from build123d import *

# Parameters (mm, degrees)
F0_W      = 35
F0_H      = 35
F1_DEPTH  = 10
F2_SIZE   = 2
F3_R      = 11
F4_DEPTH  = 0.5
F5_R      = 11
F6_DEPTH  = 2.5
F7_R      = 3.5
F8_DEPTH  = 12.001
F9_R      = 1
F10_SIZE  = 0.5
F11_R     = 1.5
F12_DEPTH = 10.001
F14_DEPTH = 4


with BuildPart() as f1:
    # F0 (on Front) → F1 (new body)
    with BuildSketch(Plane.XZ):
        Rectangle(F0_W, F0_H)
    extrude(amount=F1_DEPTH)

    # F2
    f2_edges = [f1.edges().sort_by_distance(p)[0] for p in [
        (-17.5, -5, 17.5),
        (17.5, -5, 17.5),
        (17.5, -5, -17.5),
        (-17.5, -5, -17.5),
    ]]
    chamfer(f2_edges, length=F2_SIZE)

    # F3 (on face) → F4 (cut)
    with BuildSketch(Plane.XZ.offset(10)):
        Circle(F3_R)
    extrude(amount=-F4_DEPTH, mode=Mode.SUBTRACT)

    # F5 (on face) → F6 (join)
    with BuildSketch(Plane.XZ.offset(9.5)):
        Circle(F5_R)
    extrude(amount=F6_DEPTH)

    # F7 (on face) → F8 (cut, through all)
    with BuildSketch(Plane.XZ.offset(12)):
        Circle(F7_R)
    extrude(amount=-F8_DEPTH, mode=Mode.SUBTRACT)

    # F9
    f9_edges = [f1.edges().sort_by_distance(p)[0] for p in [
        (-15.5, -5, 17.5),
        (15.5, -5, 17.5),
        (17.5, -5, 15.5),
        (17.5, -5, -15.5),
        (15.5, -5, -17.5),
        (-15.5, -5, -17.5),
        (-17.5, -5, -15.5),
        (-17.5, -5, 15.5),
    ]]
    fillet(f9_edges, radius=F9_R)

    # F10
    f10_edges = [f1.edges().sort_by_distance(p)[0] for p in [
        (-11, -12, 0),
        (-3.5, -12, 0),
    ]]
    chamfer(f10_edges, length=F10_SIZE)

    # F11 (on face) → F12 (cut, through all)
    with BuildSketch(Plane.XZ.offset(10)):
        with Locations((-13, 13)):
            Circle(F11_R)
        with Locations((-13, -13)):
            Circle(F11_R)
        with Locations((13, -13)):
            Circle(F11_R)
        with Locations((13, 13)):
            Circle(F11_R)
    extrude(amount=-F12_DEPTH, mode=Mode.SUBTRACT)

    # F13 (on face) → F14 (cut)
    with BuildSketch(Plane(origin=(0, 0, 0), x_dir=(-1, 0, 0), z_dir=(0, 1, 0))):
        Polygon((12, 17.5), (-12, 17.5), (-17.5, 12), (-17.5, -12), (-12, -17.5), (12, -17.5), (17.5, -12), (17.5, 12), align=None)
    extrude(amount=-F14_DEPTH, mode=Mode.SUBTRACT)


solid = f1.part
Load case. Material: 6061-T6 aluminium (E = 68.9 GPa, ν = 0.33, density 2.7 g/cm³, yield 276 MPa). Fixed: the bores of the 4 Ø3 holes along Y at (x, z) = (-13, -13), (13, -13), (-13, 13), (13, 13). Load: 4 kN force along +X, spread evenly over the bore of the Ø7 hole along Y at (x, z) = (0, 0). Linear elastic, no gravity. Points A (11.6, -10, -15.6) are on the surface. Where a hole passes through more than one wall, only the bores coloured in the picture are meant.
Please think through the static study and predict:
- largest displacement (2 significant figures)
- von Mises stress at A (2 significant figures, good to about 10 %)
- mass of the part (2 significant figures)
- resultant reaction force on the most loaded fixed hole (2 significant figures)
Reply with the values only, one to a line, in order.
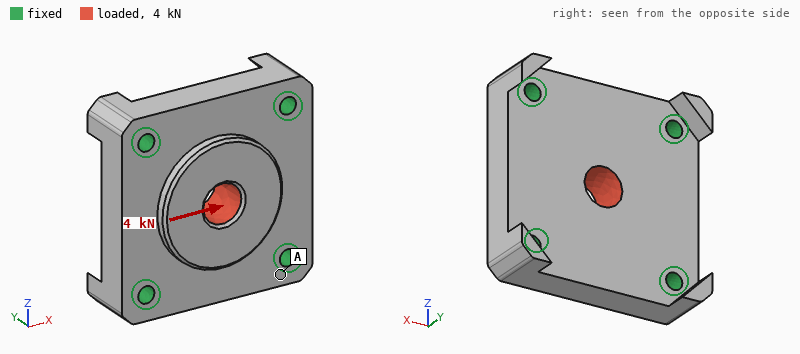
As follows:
5.9 µm
7.6 MPa
21 g
1.1 kN
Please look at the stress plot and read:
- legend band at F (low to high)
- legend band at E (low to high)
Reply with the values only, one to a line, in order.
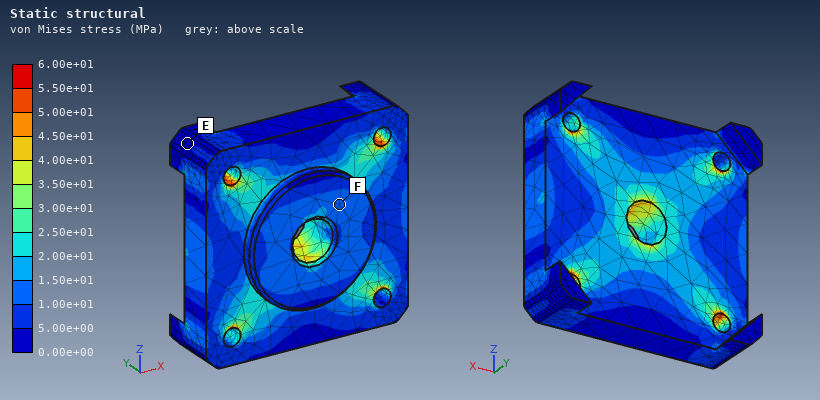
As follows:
1.00e+01 to 1.50e+01 MPa
0.00e+00 to 5.00e+00 MPa
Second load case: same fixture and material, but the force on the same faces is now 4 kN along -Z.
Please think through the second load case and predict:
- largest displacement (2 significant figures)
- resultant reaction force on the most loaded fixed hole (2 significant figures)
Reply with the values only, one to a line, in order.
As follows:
5.9 µm
1.1 kN
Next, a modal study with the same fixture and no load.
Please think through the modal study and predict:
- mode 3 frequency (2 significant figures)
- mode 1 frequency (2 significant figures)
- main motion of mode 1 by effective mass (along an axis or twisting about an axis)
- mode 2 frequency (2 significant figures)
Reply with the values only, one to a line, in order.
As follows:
38 kHz
27 kHz
along Y
38 kHz
